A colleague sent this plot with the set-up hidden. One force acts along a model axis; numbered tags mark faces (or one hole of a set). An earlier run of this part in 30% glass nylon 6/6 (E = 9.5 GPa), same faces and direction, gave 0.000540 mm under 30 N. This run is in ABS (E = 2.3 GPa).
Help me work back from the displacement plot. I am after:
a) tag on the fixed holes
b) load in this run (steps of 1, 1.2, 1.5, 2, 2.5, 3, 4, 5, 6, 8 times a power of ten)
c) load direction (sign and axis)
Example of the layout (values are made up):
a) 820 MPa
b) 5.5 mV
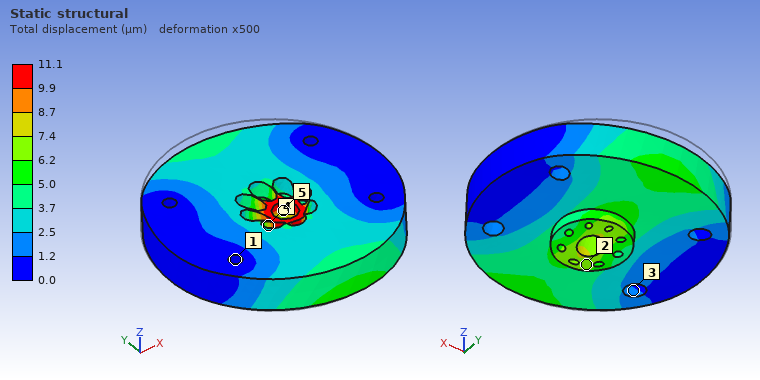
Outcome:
a) 1
b) 150 N
c) -Y
